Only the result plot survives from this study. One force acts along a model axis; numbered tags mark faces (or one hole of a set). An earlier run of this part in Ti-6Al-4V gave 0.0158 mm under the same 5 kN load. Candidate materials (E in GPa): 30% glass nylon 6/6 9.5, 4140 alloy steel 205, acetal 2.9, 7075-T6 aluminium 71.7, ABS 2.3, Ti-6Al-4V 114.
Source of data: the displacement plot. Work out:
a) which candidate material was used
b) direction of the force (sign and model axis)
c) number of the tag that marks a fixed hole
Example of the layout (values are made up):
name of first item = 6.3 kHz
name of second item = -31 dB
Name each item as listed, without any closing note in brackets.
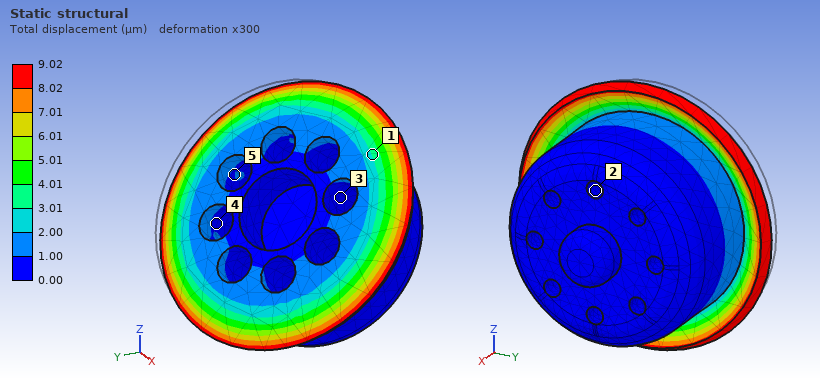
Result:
which candidate material was used = 4140 alloy steel
direction of the force = +X
number of the tag that marks a fixed hole = 2
